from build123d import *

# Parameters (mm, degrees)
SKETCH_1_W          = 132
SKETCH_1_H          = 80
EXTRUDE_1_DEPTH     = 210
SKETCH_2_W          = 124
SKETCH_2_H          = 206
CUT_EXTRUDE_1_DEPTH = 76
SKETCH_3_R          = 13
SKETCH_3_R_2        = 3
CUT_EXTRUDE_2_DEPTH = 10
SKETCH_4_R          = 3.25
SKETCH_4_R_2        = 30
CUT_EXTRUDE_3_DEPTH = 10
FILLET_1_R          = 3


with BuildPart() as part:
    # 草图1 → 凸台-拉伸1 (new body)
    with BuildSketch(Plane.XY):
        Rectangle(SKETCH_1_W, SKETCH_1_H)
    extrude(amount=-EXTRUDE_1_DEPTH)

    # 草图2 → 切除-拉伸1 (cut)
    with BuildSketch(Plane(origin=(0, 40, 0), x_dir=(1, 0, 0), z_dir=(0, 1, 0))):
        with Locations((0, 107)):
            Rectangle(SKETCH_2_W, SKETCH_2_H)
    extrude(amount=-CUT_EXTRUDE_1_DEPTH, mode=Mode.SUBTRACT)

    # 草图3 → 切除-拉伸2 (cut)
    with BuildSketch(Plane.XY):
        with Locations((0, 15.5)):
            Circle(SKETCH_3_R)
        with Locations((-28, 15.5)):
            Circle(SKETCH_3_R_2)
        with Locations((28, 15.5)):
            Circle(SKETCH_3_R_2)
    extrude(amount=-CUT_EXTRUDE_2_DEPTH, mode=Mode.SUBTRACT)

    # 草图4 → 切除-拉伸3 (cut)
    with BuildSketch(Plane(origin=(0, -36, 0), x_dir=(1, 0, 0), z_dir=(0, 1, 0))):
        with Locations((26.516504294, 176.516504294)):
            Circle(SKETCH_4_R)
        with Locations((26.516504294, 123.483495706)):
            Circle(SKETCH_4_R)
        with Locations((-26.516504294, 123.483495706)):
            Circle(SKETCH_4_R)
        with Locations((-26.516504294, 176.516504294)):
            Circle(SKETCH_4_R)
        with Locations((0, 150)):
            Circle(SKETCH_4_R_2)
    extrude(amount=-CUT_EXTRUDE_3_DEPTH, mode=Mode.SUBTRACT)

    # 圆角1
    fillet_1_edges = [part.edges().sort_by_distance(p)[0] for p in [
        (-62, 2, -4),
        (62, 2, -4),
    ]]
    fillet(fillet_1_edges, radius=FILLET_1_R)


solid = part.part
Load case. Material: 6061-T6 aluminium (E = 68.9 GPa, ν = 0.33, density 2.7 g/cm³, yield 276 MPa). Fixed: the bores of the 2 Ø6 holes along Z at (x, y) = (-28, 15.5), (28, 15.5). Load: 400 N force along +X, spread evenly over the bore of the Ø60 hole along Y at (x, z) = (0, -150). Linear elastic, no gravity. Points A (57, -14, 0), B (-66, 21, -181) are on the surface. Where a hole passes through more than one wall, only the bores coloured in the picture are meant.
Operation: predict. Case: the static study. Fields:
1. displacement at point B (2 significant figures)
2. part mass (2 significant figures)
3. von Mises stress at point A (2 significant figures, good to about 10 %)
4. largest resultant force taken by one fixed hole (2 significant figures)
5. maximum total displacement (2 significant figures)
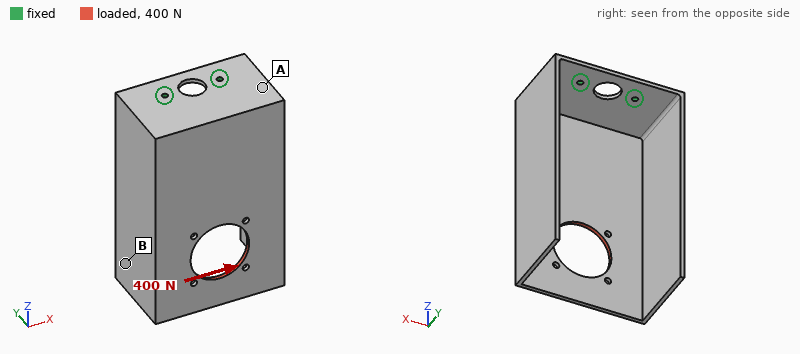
2.5 mm
710 g
16 MPa
810 N
3.0 mm
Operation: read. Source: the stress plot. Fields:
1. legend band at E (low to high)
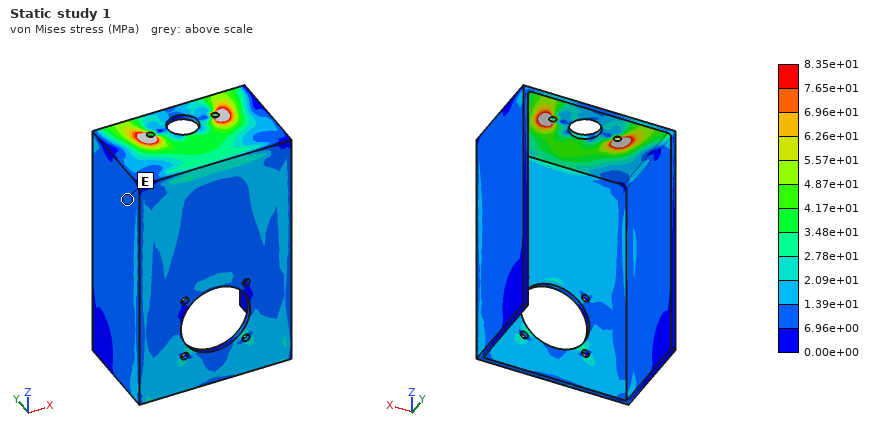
6.96e+00 to 1.39e+01 MPa
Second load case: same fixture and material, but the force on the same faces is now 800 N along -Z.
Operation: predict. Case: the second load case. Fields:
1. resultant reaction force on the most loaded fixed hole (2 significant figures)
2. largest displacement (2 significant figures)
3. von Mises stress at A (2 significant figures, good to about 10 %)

400 N
3.0 mm
21 MPa
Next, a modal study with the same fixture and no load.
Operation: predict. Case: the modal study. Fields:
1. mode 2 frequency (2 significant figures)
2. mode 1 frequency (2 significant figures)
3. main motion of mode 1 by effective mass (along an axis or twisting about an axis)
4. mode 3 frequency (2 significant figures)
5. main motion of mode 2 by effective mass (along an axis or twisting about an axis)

100 Hz
84 Hz
along Y
330 Hz
along X
